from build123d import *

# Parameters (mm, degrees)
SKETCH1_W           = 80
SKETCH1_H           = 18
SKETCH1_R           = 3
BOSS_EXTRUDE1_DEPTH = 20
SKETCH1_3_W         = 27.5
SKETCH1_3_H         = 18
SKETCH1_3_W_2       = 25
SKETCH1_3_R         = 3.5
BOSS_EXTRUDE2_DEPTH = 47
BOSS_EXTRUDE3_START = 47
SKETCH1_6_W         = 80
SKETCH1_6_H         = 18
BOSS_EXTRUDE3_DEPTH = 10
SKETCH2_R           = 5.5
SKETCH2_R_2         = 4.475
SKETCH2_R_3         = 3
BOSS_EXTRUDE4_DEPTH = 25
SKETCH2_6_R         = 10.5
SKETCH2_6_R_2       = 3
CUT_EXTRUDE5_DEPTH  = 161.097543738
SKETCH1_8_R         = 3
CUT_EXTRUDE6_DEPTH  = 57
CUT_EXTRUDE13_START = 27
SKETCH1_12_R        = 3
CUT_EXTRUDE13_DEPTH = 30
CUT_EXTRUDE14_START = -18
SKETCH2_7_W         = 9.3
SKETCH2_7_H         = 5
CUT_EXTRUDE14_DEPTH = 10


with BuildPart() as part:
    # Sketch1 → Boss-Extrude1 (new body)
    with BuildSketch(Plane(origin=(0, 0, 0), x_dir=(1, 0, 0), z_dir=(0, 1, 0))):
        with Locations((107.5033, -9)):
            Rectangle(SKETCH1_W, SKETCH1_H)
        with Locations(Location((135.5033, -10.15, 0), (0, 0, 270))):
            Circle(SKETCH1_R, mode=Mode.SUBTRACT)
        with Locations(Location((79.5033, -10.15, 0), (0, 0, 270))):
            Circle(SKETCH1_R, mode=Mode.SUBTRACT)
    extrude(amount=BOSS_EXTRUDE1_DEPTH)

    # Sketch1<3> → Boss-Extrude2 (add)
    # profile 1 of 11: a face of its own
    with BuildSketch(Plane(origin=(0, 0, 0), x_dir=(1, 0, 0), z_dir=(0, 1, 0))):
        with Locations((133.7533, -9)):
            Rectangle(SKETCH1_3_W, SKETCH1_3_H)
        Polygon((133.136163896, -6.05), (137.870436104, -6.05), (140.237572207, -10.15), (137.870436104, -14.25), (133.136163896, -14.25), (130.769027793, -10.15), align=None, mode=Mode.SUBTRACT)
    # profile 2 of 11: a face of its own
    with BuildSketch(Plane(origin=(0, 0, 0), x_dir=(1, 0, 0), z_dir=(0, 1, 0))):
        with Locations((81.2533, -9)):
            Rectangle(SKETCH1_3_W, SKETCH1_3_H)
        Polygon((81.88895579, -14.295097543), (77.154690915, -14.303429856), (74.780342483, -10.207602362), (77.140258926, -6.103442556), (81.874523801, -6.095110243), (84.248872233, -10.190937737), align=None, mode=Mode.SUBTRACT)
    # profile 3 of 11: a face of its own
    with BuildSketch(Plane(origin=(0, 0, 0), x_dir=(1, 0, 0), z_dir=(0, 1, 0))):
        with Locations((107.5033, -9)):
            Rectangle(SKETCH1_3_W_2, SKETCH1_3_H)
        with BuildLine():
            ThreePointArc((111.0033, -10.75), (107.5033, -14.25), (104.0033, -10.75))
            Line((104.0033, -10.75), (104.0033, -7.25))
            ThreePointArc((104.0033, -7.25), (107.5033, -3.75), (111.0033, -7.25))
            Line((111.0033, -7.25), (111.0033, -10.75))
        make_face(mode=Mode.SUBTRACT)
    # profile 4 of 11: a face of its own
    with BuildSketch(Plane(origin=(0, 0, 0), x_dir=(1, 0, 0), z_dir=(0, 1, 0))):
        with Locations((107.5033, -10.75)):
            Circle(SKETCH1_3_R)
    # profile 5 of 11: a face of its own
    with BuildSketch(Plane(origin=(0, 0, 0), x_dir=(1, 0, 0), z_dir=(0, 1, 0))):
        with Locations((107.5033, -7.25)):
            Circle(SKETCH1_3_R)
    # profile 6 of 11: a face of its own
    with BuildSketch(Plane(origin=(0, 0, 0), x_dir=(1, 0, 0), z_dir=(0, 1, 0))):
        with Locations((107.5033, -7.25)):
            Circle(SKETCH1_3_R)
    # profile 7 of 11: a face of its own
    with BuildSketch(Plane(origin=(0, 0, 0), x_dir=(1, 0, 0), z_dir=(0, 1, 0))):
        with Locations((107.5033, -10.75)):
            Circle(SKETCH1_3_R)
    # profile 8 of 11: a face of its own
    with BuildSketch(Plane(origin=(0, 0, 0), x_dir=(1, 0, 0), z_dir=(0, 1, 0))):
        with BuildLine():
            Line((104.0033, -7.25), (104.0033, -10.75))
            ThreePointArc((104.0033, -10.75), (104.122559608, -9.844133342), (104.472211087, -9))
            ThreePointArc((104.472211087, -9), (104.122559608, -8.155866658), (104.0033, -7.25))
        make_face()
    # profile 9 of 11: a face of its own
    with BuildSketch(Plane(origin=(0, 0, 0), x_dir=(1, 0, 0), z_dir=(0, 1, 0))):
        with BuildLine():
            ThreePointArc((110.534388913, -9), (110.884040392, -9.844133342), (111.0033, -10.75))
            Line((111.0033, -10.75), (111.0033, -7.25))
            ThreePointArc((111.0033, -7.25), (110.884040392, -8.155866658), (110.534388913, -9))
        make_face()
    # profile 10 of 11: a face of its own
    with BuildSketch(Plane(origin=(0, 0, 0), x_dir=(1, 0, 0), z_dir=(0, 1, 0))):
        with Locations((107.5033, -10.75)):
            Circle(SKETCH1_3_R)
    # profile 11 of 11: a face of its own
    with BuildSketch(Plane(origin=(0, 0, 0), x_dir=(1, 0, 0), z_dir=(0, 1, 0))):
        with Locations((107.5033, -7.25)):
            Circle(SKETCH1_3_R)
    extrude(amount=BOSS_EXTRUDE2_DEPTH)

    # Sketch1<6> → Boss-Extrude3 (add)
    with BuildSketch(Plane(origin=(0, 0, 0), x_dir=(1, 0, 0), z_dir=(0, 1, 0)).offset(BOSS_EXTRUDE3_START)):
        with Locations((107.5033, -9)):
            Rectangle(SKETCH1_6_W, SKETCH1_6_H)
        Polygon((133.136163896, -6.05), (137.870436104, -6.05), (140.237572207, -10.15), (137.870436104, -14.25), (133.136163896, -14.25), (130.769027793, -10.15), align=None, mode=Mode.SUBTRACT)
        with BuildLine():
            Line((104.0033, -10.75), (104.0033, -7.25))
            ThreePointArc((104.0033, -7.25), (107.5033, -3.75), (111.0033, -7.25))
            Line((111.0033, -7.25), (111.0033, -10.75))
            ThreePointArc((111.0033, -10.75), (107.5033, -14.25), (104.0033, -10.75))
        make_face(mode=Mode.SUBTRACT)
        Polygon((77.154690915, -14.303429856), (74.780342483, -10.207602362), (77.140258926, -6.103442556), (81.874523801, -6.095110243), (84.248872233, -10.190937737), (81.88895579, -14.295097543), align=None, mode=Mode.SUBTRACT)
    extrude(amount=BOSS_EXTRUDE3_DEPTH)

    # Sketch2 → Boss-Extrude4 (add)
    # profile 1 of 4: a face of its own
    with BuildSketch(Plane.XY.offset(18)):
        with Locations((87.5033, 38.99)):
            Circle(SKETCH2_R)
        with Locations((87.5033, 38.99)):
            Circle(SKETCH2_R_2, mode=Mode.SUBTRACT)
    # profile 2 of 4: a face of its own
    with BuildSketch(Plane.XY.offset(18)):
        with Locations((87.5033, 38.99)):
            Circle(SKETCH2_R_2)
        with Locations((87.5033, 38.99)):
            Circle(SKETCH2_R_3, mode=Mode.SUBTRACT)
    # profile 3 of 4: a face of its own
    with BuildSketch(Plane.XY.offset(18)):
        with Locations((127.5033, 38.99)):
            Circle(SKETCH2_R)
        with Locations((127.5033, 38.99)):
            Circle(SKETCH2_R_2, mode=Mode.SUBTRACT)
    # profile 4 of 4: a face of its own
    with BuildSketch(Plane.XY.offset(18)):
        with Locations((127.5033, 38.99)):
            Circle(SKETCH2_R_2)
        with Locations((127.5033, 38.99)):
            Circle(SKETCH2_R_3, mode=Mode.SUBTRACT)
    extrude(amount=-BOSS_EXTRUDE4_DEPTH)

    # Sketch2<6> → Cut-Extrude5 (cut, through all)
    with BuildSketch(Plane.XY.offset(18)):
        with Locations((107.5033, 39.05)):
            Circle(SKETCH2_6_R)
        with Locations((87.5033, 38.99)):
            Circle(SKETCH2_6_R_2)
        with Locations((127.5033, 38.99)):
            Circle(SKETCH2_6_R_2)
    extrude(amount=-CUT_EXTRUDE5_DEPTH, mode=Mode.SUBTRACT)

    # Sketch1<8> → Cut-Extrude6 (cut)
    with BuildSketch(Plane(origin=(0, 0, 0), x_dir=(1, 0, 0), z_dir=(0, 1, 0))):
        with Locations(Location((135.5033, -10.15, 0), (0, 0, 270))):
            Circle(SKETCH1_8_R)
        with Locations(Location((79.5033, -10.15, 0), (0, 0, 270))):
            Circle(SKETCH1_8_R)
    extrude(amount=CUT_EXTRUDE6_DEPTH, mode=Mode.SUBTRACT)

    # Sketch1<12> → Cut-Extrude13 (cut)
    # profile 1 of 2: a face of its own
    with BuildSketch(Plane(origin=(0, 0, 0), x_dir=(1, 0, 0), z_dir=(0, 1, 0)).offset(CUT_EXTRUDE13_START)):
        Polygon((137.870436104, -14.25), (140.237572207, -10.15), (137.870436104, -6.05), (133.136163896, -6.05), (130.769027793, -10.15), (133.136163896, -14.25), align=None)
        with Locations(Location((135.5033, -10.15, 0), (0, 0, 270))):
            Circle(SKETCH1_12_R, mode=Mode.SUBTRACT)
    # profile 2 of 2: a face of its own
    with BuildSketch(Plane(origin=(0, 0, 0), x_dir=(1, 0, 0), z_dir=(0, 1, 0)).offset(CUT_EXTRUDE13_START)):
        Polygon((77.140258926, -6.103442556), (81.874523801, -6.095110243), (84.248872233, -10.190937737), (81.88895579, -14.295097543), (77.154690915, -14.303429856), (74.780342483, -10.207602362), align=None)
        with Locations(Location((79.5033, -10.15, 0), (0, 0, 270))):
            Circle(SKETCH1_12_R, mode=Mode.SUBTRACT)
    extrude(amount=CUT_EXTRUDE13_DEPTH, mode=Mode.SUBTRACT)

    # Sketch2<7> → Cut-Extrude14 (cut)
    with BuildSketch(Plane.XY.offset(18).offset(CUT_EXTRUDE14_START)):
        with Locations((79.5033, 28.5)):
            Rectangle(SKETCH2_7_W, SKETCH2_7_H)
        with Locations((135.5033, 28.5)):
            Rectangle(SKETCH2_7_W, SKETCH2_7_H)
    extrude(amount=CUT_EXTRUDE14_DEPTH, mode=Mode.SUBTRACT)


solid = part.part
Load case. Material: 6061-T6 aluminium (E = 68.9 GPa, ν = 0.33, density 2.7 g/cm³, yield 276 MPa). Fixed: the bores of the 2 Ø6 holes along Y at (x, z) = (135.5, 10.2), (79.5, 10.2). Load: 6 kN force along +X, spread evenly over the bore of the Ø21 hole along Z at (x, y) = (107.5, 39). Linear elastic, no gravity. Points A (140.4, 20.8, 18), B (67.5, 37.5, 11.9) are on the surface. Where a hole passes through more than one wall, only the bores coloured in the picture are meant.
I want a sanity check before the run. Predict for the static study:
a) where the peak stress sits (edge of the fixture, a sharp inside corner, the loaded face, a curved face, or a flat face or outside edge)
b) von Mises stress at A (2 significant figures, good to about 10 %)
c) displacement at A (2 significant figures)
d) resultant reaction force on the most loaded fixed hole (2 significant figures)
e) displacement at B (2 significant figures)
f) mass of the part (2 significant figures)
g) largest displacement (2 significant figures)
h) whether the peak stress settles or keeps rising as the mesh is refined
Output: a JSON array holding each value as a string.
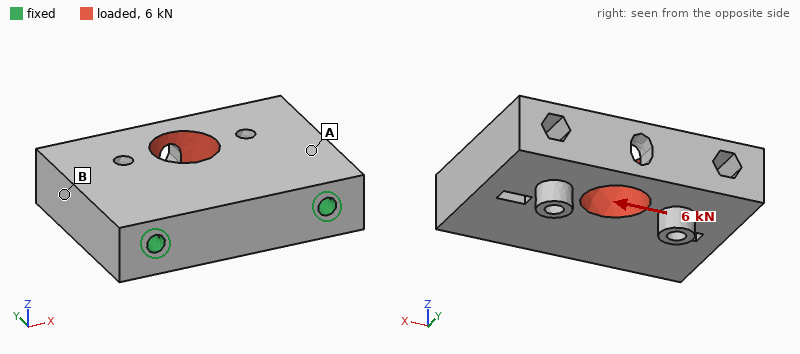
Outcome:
["edge of the fixture", "7.9 MPa", "2.5 µm", "3.8 kN", "9.2 µm", "190 g", "15 µm", "keeps rising"]
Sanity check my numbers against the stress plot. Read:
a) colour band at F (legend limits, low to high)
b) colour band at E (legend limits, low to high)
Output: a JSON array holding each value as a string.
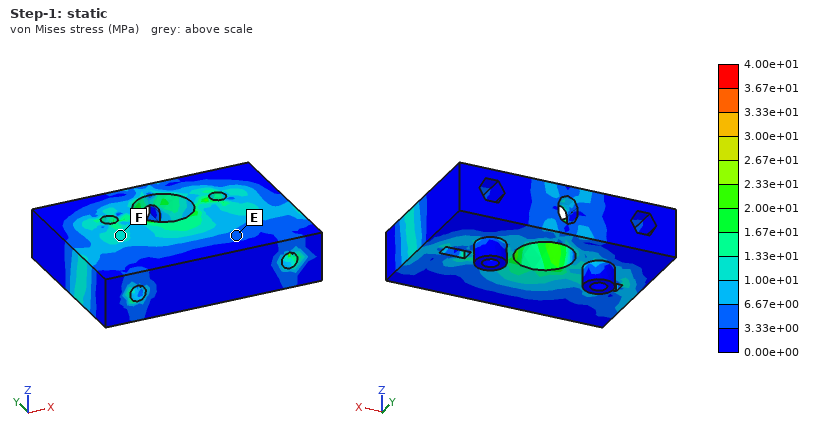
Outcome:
["1.00e+01 to 1.33e+01 MPa", "3.33e+00 to 6.67e+00 MPa"]
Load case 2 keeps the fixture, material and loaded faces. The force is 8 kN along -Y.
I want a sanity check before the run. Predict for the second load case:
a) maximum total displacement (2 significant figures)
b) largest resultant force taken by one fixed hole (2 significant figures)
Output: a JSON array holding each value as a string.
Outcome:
["13 µm", "4.3 kN"]
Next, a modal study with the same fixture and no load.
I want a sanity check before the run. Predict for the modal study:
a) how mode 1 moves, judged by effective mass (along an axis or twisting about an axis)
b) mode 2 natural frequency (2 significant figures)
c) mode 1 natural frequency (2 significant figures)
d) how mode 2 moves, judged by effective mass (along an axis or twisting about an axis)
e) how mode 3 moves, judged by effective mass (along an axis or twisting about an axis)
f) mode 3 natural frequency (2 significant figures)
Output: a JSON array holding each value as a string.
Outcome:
["along Z", "8100 Hz", "5000 Hz", "twisting about Y", "along X", "11 kHz"]
